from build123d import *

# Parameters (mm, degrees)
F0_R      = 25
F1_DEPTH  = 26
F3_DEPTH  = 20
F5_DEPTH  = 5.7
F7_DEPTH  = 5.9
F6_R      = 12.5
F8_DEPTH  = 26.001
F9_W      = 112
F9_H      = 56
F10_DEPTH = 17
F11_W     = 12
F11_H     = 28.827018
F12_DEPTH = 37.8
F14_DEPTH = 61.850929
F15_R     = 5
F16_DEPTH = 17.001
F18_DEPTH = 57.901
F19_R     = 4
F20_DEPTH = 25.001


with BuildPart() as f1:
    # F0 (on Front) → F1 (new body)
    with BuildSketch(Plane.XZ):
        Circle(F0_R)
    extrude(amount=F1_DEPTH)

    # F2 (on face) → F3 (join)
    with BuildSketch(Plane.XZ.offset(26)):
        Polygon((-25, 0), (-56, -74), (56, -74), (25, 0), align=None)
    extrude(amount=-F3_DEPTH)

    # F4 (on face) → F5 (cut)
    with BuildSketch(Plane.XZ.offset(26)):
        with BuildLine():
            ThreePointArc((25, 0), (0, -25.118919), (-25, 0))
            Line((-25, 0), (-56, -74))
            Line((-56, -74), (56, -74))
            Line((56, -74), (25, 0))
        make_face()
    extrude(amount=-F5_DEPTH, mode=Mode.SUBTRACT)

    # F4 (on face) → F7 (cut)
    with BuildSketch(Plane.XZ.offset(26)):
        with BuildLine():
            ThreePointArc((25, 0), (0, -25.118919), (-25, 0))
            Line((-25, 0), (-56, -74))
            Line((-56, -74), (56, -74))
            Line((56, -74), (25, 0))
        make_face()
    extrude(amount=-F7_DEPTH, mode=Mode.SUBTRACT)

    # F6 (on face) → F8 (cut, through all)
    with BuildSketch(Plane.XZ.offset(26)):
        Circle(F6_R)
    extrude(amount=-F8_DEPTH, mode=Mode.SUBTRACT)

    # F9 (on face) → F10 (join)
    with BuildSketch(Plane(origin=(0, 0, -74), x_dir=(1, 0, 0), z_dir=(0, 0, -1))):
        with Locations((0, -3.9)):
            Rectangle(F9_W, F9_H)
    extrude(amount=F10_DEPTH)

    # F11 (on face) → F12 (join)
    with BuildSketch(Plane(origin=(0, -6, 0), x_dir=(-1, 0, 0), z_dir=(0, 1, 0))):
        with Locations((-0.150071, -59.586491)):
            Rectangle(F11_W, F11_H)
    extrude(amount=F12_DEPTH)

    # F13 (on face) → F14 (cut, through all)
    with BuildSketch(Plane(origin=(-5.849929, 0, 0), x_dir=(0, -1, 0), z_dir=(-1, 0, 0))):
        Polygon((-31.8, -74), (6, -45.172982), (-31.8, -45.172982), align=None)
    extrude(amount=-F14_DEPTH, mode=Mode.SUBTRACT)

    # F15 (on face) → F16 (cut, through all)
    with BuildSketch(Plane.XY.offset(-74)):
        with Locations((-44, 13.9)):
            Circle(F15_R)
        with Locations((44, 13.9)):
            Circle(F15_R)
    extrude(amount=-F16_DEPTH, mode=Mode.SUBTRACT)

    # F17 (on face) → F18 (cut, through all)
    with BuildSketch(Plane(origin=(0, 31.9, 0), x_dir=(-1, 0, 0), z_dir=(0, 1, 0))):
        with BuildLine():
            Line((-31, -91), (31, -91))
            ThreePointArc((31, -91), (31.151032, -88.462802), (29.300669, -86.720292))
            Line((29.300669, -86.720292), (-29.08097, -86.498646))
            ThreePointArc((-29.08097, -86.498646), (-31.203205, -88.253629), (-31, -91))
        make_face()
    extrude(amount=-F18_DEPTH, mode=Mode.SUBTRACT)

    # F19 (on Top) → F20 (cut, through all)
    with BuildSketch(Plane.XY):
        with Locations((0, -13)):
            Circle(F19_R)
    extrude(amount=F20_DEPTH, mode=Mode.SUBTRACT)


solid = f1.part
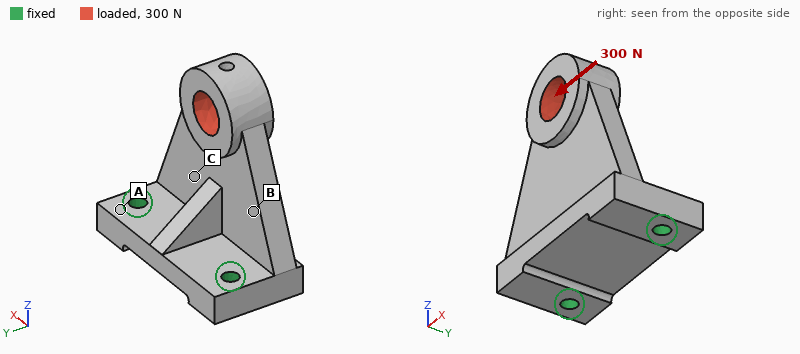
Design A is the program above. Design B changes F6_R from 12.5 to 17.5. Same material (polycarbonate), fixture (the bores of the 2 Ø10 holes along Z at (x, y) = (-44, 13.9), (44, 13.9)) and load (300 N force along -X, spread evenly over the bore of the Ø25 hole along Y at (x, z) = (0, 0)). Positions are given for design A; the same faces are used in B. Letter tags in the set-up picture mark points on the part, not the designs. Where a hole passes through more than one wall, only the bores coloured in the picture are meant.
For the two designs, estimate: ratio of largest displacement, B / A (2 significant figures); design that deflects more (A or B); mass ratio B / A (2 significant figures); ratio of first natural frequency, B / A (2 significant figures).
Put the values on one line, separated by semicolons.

1.2; B; 0.94; 1.1
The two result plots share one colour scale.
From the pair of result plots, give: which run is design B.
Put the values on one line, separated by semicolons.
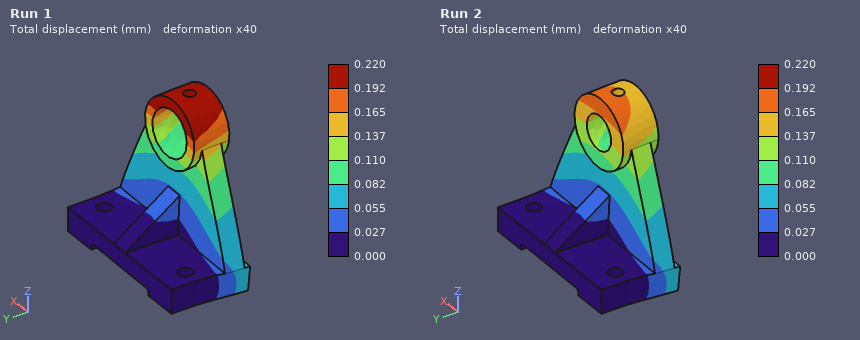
Run 1
